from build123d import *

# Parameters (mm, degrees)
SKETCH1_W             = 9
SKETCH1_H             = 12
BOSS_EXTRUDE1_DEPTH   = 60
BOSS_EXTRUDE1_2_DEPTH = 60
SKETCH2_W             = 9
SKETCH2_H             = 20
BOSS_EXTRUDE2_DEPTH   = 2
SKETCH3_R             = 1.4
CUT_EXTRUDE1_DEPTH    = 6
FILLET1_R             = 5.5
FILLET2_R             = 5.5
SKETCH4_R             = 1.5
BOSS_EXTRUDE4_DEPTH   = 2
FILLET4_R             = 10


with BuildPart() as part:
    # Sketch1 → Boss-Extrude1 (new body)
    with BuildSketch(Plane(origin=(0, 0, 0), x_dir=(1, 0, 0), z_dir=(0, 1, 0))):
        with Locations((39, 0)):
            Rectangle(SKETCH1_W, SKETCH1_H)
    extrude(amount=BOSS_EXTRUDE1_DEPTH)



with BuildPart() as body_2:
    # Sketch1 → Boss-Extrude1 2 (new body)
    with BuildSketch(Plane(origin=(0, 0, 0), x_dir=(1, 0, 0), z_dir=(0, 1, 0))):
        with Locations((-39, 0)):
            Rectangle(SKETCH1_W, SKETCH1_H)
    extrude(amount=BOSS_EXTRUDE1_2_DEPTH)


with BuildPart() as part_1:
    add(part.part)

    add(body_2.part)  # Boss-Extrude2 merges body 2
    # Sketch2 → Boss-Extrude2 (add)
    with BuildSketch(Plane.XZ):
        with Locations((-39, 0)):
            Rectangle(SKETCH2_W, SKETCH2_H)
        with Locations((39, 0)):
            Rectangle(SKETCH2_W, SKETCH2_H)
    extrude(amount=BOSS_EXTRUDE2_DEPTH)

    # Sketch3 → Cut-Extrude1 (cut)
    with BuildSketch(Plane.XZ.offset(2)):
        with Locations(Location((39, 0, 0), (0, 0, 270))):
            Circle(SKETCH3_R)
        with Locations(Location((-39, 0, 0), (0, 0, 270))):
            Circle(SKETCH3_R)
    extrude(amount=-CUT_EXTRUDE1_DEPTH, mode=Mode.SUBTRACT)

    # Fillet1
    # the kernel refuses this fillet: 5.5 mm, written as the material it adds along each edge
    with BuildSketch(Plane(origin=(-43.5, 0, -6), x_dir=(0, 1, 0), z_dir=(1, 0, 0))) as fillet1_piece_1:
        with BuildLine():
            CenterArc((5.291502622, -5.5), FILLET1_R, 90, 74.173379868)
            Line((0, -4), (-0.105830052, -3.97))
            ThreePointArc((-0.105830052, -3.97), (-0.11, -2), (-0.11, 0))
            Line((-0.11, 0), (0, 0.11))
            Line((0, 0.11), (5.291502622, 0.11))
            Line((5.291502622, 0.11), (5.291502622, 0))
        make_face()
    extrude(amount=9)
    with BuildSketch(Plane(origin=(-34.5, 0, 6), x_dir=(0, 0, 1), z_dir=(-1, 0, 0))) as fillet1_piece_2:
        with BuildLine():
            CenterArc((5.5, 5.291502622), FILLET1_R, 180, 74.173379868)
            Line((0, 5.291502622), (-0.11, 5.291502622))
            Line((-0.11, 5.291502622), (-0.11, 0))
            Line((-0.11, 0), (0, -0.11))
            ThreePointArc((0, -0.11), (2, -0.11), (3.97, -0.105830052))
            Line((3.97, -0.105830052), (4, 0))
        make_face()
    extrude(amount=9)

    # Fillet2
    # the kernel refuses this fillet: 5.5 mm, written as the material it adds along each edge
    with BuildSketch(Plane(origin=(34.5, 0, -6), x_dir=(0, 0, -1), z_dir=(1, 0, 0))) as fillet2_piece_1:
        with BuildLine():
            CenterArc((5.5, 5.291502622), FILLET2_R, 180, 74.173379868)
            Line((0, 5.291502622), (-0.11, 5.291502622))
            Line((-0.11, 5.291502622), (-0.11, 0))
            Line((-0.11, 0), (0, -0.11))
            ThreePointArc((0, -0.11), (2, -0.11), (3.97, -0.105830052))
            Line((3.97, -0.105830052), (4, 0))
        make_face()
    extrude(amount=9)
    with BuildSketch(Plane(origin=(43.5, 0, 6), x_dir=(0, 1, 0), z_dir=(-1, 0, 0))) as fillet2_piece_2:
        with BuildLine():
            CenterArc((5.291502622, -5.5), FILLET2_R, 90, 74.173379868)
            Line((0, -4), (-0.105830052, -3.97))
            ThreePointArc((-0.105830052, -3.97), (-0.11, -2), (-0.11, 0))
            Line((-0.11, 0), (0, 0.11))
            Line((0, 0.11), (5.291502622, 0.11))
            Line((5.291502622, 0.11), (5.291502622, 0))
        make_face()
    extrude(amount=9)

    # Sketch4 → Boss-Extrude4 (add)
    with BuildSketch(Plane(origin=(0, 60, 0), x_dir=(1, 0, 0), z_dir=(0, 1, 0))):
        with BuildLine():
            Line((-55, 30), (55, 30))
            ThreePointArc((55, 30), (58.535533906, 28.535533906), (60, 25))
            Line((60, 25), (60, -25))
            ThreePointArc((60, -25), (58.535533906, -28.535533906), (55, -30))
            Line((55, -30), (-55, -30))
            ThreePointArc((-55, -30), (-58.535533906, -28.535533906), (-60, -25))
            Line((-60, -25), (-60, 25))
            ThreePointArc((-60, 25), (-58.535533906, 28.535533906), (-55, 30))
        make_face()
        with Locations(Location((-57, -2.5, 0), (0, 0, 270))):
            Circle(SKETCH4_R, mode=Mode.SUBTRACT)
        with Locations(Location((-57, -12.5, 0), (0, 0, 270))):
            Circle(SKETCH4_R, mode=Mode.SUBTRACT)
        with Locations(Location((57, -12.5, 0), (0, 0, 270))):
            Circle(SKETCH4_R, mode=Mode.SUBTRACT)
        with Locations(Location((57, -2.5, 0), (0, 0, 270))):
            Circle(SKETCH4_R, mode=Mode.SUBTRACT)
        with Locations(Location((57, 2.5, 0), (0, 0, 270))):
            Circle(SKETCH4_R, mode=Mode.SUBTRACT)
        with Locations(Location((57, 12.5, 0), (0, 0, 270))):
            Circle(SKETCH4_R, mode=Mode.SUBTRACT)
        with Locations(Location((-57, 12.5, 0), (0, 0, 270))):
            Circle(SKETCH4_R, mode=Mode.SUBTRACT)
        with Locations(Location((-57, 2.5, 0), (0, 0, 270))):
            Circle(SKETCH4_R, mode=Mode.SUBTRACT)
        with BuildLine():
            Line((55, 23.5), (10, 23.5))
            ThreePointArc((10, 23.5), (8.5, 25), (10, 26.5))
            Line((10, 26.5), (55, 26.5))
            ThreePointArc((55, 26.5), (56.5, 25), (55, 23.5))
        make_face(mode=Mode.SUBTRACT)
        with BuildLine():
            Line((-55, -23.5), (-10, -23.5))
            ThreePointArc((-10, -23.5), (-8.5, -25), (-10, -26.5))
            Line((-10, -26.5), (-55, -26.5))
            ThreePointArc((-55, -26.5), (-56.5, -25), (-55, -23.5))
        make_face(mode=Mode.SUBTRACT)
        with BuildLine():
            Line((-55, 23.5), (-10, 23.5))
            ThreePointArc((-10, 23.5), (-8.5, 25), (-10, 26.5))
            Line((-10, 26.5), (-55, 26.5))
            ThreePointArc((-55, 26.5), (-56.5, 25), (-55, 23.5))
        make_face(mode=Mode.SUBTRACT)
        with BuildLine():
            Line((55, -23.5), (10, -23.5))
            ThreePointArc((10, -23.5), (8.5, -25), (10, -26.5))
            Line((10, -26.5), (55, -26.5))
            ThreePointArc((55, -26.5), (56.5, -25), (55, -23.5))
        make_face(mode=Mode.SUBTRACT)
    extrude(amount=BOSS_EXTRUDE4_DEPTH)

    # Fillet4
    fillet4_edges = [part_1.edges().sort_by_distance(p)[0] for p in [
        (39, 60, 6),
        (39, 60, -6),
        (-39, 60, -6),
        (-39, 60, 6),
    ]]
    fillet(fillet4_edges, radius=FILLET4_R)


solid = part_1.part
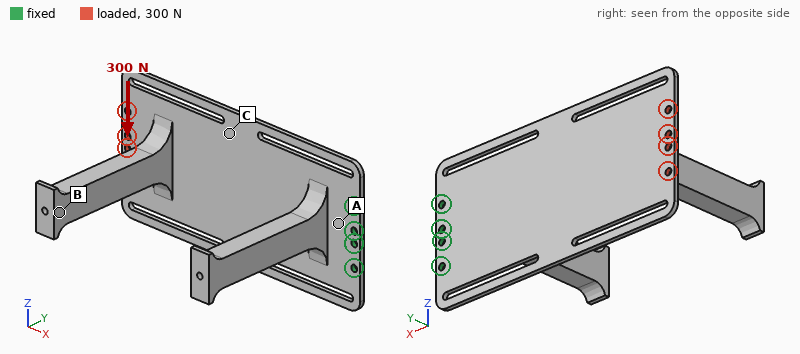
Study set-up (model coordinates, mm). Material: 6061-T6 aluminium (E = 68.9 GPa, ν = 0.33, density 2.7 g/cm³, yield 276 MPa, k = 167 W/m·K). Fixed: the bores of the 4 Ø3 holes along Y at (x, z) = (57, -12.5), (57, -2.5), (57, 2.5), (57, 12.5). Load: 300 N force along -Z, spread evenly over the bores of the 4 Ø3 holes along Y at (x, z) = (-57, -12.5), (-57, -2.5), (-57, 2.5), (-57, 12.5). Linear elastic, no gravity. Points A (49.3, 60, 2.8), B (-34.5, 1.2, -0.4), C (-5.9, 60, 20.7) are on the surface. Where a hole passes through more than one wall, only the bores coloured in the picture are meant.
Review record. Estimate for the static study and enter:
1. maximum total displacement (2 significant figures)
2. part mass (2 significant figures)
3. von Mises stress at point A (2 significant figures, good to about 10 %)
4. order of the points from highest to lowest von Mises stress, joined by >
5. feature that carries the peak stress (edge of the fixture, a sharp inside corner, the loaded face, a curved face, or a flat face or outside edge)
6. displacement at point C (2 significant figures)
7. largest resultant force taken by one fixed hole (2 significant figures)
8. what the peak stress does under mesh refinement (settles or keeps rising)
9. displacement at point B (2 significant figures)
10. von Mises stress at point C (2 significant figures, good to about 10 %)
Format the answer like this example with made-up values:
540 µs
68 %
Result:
0.19 mm
75 g
25 MPa
A > C > B
edge of the fixture
0.088 mm
1.2 kN
keeps rising
0.10 mm
14 MPa
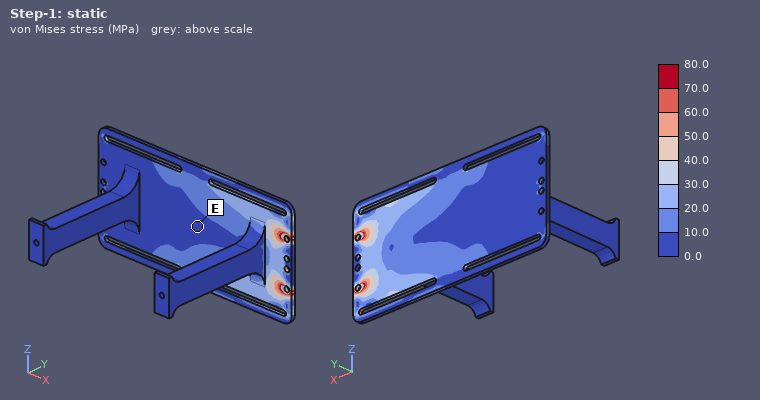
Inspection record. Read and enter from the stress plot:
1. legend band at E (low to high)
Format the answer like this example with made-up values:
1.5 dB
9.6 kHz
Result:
0.0 to 10.0 MPa
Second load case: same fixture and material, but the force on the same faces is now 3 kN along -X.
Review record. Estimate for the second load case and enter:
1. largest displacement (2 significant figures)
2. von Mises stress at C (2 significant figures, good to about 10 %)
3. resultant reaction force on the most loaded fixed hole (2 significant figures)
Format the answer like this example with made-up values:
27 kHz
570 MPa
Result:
0.16 mm
28 MPa
940 N
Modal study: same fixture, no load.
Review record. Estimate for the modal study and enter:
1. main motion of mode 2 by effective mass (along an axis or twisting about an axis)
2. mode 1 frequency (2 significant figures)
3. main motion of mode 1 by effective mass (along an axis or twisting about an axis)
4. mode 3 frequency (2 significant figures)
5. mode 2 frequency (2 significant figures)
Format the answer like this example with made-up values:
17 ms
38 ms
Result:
along Z
76 Hz
along Y
300 Hz
210 Hz
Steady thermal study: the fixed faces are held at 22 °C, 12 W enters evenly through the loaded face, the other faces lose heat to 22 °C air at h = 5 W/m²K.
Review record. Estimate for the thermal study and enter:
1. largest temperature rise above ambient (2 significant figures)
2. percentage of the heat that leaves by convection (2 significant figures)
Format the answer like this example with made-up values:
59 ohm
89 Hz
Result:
68 K
25 %
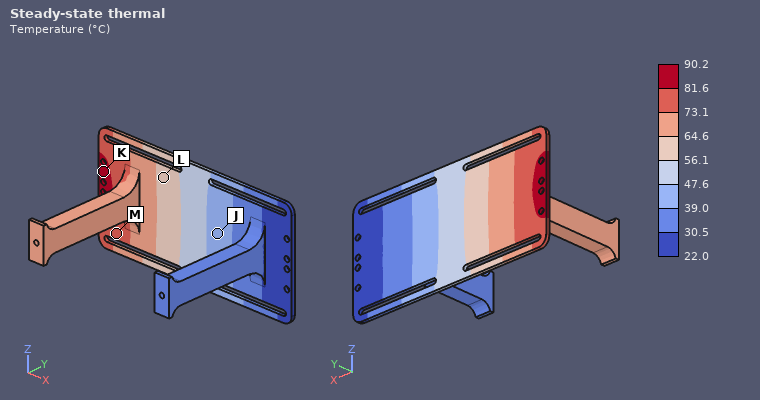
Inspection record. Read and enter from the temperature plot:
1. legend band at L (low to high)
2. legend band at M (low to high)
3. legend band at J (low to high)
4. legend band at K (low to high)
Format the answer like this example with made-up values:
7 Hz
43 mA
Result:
56.1 to 64.6 °C
73.1 to 81.6 °C
39.0 to 47.6 °C
81.6 to 90.2 °C
